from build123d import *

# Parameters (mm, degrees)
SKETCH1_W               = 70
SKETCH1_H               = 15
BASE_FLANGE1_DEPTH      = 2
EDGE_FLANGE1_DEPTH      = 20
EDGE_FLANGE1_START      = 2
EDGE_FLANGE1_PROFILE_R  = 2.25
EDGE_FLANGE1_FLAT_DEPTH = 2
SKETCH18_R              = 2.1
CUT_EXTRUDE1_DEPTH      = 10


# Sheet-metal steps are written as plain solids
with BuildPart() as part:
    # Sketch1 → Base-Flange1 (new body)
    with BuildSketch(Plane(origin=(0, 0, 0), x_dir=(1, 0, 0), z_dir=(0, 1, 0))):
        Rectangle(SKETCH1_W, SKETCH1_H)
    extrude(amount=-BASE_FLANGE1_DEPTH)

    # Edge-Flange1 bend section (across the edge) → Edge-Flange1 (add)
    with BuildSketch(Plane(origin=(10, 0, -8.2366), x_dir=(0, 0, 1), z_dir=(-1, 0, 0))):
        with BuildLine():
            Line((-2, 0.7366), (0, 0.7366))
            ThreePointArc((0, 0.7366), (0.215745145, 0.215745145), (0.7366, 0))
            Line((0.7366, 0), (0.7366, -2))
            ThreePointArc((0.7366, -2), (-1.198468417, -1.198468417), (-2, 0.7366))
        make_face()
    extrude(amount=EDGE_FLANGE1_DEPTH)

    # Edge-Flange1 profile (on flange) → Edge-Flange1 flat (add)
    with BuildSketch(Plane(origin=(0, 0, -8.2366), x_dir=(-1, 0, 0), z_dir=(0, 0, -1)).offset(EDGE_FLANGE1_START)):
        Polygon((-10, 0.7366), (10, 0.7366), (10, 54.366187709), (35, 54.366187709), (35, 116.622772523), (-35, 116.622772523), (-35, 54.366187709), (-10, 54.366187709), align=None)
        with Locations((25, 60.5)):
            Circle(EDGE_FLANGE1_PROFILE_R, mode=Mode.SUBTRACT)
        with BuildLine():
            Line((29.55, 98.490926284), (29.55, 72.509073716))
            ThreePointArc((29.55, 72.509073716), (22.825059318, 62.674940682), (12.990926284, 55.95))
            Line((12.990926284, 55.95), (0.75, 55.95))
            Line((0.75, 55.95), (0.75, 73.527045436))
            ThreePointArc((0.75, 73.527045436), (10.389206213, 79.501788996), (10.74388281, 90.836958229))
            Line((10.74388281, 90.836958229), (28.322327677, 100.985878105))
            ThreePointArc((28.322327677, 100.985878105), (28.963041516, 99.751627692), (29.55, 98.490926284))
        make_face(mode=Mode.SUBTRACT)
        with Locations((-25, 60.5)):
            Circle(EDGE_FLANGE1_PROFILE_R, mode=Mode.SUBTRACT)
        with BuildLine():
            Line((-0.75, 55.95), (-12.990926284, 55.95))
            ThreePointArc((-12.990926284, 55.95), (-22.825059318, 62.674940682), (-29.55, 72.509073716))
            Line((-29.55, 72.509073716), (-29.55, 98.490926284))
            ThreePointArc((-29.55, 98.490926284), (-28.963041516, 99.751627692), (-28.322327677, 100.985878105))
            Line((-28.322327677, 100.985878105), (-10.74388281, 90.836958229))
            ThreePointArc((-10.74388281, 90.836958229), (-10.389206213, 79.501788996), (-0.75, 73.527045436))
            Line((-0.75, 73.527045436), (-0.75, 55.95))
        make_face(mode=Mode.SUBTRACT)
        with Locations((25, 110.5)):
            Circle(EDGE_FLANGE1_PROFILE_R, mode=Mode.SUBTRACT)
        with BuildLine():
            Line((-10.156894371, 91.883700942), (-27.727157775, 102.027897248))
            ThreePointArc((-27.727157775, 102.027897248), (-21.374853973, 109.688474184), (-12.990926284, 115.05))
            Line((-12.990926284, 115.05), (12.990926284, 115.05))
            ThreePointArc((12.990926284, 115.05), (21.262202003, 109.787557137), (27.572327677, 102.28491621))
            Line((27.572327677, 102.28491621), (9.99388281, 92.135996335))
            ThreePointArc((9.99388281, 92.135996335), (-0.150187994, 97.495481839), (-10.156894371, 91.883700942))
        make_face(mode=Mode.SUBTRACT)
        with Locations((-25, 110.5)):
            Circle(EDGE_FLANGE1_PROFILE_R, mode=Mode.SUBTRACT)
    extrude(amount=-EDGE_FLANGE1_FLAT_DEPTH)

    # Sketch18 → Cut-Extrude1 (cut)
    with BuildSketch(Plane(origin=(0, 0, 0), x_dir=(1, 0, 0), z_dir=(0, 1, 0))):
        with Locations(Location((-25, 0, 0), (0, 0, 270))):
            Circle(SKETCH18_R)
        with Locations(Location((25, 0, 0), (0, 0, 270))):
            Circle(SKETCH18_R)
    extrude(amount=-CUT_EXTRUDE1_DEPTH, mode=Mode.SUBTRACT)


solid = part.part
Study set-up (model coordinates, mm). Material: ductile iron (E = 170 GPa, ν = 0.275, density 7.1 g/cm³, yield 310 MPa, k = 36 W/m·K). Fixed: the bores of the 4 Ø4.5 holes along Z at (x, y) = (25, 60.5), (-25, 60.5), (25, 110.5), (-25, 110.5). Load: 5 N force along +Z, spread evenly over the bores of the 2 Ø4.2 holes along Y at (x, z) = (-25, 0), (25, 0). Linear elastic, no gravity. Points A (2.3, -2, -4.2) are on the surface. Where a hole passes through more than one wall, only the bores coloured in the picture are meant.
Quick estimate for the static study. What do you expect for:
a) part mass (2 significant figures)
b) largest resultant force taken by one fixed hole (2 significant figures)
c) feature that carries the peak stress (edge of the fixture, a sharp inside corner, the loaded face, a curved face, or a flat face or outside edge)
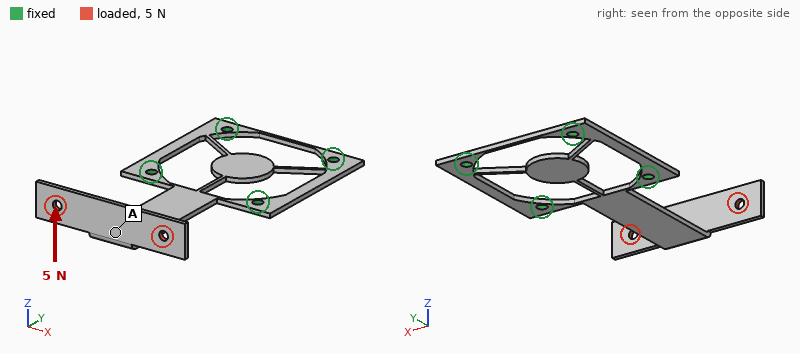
55 g
3.5 N
a flat face or outside edge
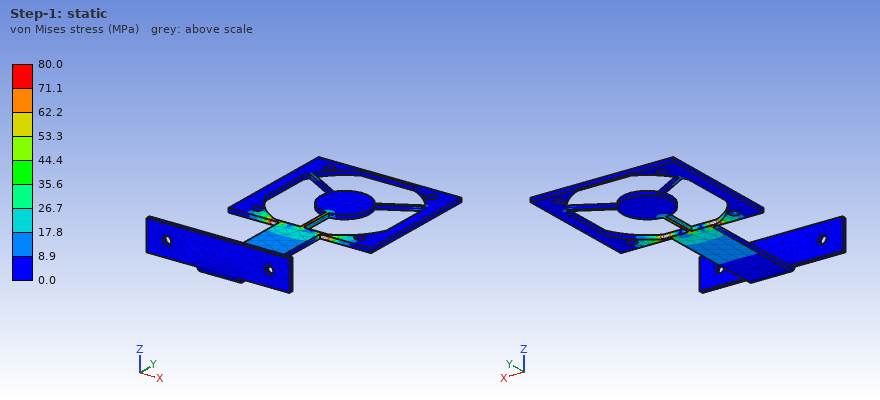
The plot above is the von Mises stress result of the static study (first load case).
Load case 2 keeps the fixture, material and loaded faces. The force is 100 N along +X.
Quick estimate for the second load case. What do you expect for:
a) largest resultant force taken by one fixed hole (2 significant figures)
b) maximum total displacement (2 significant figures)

250 N
0.85 mm
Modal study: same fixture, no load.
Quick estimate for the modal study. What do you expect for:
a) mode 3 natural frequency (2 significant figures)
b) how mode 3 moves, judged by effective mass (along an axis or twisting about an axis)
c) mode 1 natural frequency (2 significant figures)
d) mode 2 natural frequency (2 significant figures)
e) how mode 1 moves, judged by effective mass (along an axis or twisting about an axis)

660 Hz
along X
110 Hz
410 Hz
along Z
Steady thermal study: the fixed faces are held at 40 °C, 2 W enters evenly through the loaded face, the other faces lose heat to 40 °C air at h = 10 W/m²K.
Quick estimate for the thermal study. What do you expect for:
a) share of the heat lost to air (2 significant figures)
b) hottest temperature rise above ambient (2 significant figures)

84 %
52 K
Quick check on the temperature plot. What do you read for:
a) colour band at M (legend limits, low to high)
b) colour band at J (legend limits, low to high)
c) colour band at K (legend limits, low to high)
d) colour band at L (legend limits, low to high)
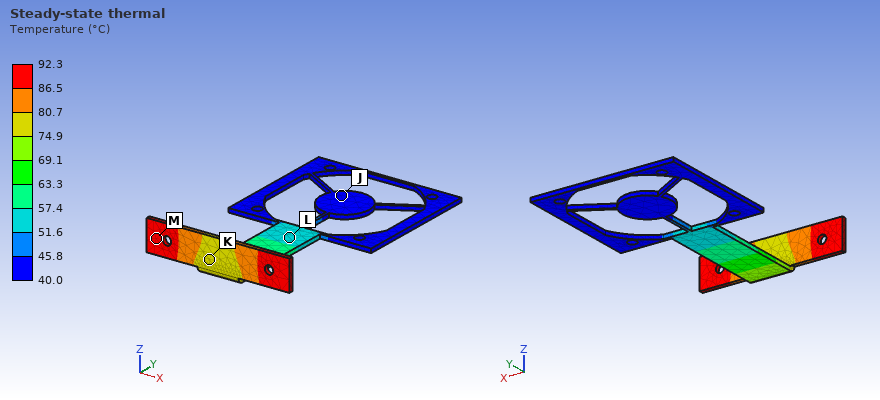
86.5 to 92.3 °C
40.0 to 45.8 °C
74.9 to 80.7 °C
51.6 to 57.4 °C
